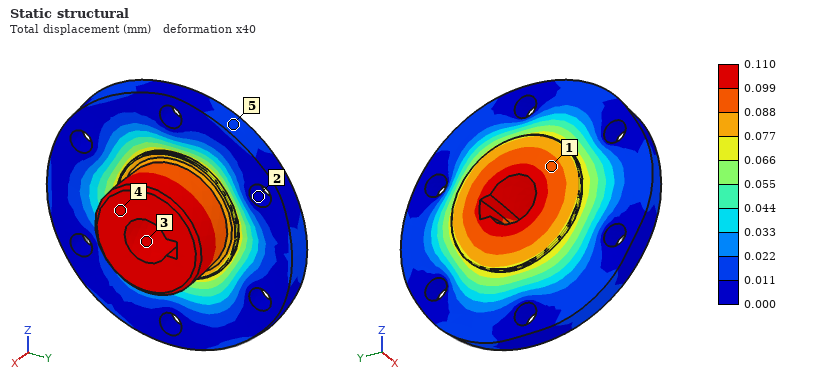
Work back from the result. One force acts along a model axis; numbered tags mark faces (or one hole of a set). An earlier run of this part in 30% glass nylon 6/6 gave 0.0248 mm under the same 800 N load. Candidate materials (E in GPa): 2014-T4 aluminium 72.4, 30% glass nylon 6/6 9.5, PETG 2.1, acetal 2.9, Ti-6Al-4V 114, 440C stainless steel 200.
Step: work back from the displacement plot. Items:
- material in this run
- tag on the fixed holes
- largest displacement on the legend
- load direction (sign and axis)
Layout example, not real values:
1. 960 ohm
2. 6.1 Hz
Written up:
1. PETG
2. 2
3. 0.110 mm
4. -X
